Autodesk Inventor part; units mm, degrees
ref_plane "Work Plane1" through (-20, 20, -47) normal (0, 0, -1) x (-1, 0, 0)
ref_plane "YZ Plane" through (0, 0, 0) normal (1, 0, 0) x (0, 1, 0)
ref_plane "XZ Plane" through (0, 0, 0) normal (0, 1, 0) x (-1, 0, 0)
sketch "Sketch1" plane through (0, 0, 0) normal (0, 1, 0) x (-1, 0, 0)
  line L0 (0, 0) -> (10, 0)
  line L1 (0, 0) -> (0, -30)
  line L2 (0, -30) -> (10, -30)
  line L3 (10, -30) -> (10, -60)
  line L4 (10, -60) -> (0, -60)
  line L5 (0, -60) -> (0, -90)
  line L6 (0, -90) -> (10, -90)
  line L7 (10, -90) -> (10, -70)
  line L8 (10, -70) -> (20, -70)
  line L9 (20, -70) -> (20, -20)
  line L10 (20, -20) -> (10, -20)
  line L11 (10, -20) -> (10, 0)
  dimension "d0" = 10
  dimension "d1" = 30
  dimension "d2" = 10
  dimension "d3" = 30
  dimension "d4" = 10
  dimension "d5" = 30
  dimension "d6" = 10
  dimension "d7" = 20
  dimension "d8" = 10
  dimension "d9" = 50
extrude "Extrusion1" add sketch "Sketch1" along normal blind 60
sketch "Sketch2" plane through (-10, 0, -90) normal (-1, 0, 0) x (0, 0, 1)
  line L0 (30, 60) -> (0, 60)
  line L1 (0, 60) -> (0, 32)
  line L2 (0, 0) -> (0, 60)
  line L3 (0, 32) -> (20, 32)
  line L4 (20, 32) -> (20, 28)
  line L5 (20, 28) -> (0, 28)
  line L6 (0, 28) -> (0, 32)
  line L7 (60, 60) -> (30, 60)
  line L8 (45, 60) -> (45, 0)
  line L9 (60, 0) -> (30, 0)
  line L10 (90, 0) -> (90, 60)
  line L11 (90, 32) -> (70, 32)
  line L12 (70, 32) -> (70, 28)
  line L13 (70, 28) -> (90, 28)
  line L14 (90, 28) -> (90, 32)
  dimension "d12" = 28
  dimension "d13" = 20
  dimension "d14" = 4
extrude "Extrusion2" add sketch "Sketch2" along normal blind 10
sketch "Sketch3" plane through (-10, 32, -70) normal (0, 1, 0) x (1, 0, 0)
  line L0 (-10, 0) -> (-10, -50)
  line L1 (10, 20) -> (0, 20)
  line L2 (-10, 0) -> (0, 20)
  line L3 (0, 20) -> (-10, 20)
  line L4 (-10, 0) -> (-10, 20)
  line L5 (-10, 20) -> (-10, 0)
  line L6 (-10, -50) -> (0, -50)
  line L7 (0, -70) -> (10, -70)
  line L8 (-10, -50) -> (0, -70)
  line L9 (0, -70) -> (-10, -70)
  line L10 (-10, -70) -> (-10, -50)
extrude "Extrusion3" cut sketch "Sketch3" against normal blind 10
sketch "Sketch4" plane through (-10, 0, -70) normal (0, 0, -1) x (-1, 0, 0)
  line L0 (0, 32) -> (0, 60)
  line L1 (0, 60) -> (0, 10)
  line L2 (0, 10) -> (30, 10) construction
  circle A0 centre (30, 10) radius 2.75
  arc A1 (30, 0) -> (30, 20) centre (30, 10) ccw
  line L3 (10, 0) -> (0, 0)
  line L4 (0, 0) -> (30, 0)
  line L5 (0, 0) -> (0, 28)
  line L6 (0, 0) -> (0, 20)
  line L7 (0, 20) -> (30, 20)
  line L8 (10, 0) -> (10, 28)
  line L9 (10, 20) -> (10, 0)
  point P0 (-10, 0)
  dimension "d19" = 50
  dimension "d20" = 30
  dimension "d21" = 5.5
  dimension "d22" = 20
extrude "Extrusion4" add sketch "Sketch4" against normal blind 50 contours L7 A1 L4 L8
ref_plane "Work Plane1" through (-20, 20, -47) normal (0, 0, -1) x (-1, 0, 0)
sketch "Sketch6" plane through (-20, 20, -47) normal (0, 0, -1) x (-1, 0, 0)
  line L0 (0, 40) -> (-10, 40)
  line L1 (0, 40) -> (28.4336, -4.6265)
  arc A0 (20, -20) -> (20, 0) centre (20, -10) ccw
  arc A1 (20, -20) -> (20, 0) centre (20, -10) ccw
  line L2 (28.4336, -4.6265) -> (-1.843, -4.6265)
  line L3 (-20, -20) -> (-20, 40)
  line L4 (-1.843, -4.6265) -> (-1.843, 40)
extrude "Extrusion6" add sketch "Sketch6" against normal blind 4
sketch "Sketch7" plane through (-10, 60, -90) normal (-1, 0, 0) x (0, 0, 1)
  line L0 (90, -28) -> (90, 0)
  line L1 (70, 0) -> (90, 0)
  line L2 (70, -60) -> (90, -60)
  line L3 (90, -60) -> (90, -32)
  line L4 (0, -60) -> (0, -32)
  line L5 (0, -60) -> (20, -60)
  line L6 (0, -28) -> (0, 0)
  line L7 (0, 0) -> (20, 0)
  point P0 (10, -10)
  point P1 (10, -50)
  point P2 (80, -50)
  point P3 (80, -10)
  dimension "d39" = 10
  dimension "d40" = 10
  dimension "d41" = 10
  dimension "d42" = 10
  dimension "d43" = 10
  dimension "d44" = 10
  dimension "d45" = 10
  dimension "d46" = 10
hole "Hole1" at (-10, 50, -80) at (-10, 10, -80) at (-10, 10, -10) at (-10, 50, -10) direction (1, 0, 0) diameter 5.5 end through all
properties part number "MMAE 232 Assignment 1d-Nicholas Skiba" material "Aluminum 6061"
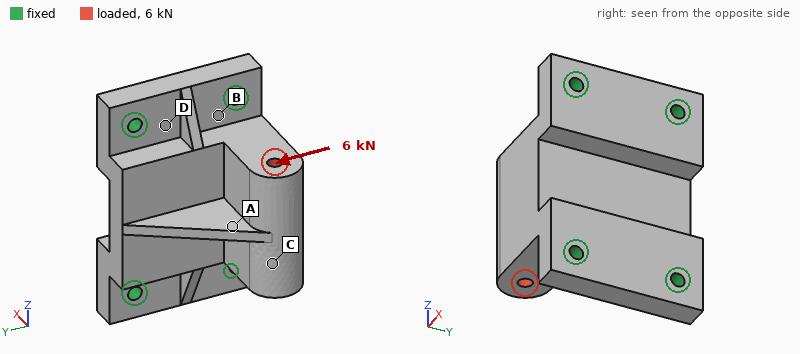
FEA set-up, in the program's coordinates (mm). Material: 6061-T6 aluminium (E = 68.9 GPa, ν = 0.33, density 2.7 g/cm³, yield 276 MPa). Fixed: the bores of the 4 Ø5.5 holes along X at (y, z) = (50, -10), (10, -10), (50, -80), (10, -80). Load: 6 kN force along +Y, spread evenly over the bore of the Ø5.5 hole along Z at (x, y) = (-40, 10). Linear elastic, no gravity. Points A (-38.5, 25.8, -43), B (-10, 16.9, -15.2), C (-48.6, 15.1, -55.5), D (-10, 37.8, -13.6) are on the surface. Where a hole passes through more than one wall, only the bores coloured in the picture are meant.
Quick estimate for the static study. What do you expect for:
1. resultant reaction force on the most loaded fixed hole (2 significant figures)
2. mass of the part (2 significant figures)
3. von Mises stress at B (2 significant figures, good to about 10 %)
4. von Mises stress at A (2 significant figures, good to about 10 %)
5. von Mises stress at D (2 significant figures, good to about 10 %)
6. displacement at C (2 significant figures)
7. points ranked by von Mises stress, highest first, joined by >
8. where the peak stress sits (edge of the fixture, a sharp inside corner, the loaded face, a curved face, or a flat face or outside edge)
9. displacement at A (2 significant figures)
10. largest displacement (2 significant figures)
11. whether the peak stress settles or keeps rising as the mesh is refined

4.2 kN
260 g
32 MPa
46 MPa
22 MPa
72 µm
A > B > D > C
edge of the fixture
49 µm
77 µm
keeps rising
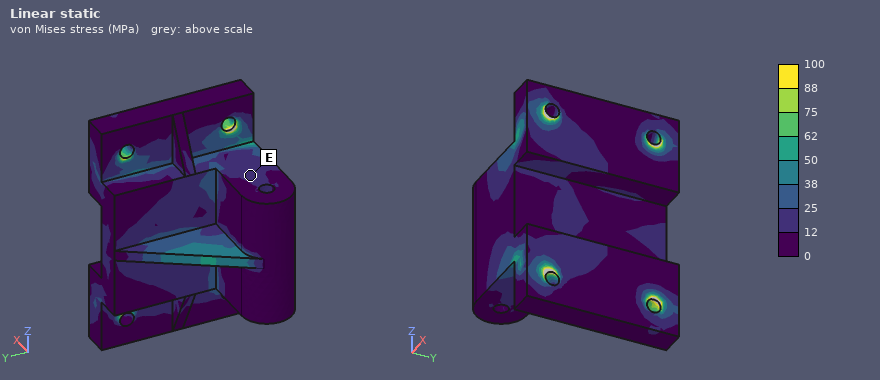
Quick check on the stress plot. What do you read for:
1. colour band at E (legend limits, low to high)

12 to 25 MPa
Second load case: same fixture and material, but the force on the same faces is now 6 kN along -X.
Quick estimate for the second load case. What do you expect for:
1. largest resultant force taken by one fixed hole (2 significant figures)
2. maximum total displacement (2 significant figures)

3.5 kN
27 µm
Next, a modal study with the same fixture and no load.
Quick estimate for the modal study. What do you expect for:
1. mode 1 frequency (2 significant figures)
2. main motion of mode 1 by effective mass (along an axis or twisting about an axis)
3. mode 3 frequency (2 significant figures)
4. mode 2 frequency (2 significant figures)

6000 Hz
along Y
9100 Hz
9000 Hz
